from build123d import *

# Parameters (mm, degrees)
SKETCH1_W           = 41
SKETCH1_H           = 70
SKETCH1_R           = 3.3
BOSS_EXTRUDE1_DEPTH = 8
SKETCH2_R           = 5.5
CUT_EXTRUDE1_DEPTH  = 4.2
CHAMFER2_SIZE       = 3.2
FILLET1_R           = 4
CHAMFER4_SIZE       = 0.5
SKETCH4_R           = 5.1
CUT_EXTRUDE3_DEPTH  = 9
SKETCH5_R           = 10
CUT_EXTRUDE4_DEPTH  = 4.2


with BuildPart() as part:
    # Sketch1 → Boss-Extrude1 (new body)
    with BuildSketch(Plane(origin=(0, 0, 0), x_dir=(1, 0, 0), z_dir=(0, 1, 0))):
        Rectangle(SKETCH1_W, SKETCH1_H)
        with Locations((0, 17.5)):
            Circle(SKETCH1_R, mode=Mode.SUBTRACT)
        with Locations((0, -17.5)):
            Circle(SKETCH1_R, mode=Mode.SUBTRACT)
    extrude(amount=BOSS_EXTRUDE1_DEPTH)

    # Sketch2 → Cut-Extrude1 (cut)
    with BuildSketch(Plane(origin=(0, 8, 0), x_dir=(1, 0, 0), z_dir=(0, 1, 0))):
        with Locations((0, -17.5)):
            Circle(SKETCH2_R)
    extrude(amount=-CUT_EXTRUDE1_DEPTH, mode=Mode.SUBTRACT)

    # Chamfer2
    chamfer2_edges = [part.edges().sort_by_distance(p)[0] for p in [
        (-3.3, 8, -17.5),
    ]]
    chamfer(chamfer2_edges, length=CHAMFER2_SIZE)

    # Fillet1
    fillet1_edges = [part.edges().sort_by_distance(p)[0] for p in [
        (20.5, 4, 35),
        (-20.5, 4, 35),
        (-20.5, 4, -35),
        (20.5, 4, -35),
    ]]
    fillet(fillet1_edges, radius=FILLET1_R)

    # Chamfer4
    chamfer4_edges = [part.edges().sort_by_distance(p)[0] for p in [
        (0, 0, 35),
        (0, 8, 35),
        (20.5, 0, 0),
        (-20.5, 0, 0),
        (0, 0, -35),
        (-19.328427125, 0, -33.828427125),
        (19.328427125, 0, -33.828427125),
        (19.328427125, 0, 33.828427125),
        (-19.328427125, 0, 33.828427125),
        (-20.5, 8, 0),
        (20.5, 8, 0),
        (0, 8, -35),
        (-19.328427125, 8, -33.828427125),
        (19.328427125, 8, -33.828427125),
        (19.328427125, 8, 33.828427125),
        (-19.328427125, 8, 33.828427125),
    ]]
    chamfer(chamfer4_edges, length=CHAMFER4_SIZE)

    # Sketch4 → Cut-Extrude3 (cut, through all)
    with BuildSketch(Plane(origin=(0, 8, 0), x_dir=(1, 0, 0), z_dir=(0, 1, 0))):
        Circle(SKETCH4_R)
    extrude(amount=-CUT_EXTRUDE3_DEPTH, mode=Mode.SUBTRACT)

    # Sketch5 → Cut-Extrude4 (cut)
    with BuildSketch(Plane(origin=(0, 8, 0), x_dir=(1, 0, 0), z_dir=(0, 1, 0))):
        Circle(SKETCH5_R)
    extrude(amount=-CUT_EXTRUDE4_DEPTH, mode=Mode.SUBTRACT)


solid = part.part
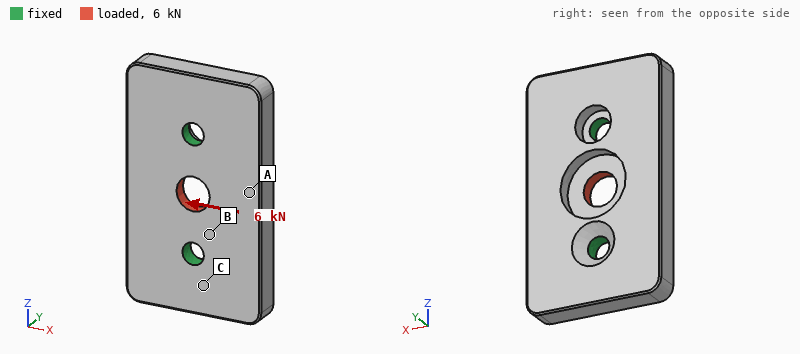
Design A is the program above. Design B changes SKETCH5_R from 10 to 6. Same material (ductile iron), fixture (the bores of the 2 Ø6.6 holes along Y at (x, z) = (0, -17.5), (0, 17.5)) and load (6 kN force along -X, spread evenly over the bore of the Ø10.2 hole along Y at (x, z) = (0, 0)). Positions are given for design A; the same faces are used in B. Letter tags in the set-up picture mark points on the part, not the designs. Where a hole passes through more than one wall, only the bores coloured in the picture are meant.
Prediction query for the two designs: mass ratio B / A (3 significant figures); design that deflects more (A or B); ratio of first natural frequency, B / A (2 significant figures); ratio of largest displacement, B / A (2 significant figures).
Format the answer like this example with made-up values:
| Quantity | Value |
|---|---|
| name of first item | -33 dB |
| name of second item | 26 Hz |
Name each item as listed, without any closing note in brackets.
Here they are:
| Quantity | Value |
|---|---|
| mass ratio B / A | 1.04 |
| design that deflects more | A |
| ratio of first natural frequency, B / A | 1.0 |
| ratio of largest displacement, B / A | 0.90 |
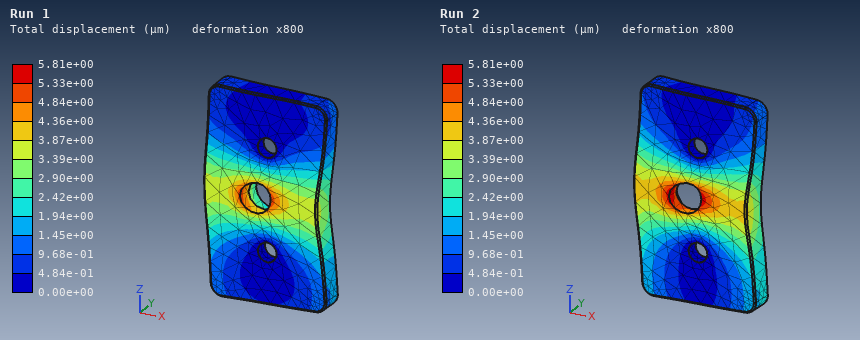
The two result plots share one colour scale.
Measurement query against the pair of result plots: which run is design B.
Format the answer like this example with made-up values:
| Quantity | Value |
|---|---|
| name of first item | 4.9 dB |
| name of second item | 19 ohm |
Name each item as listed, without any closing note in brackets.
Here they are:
| Quantity | Value |
|---|---|
| which run is design B | Run 1 |
